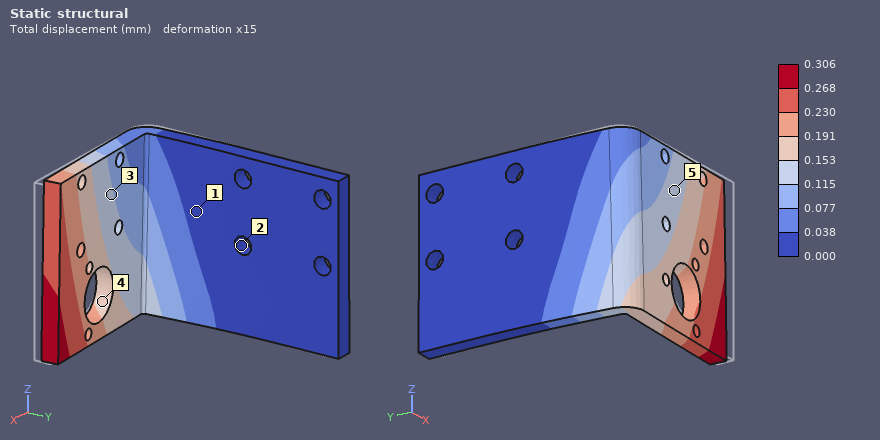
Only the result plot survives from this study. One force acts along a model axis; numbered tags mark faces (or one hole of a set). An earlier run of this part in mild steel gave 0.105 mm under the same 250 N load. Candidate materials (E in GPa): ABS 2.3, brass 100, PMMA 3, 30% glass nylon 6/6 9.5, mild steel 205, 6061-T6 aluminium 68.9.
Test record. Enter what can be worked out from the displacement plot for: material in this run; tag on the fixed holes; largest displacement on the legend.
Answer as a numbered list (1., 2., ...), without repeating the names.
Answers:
1. 6061-T6 aluminium
2. 2
3. 0.306 mm
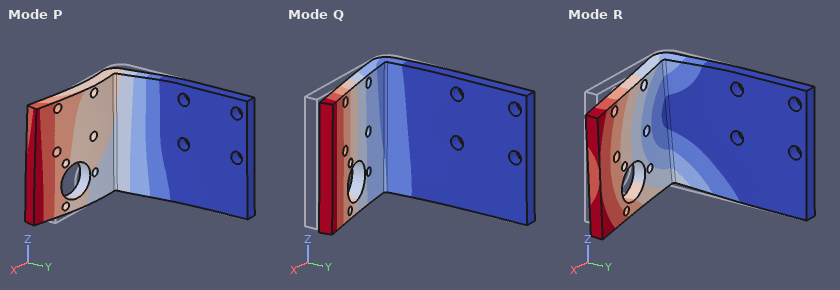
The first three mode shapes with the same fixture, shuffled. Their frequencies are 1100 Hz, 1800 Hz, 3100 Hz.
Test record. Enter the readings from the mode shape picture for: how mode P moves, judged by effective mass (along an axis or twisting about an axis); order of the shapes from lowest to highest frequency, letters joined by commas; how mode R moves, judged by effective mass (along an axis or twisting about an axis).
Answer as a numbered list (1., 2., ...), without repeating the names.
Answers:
1. along X
2. Q, R, P
3. along Z
